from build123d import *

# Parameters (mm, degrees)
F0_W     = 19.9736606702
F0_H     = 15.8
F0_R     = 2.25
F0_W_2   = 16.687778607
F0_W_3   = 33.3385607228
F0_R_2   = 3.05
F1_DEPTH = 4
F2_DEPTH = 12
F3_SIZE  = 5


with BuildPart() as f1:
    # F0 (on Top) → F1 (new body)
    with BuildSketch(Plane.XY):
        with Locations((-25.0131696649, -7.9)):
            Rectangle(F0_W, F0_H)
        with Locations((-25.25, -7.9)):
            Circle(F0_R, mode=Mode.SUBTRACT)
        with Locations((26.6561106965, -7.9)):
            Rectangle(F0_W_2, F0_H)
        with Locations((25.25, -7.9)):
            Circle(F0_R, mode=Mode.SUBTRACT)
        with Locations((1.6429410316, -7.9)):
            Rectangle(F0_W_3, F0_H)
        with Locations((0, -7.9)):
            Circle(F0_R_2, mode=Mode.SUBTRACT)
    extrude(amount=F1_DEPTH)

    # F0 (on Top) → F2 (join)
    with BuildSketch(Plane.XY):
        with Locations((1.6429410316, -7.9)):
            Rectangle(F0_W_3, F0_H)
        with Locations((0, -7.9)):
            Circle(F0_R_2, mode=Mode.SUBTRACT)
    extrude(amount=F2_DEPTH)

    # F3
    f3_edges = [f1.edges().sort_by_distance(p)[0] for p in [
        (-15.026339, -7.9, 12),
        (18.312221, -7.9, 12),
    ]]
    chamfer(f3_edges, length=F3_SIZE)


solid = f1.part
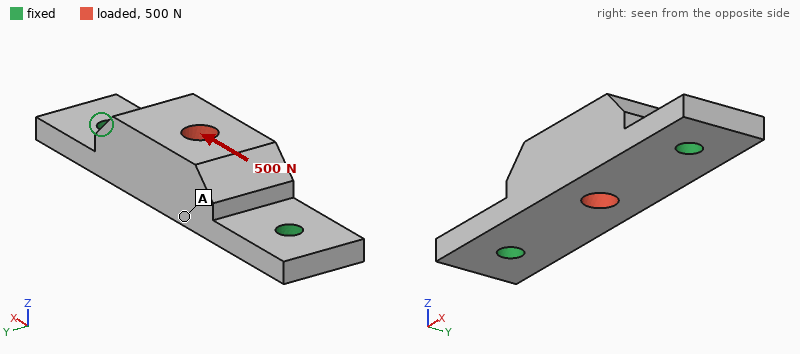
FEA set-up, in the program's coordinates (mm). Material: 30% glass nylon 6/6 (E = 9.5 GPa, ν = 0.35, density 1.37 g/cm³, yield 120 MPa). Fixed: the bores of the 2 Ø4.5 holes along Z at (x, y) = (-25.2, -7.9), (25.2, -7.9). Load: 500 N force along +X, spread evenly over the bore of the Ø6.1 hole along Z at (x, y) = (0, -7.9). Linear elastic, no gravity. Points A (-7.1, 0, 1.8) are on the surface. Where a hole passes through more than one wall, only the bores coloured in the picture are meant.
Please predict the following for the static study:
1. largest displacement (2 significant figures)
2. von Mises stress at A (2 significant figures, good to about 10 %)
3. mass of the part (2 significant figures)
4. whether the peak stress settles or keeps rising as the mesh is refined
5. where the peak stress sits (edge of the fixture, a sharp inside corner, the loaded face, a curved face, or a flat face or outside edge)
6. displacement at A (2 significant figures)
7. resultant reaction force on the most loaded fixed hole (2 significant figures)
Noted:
11 µm
1.5 MPa
11 g
keeps rising
edge of the fixture
7.8 µm
260 N
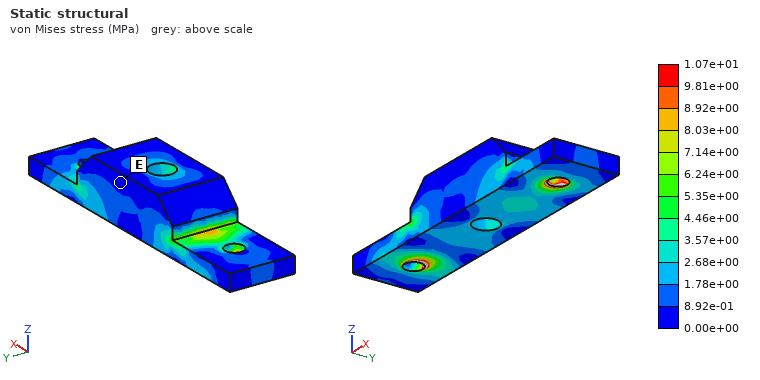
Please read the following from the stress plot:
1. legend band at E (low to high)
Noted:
0.00e+00 to 8.92e-01 MPa
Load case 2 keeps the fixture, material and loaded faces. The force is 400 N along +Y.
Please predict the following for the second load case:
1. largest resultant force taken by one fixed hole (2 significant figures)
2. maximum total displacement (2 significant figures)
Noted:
200 N
98 µm
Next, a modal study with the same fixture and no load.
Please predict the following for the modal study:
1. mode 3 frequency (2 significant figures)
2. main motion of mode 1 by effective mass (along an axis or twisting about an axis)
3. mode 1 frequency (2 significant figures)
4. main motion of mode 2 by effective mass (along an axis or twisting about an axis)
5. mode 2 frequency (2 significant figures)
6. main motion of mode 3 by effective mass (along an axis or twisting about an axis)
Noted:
8900 Hz
along Y
4200 Hz
along Z
5500 Hz
along Y
